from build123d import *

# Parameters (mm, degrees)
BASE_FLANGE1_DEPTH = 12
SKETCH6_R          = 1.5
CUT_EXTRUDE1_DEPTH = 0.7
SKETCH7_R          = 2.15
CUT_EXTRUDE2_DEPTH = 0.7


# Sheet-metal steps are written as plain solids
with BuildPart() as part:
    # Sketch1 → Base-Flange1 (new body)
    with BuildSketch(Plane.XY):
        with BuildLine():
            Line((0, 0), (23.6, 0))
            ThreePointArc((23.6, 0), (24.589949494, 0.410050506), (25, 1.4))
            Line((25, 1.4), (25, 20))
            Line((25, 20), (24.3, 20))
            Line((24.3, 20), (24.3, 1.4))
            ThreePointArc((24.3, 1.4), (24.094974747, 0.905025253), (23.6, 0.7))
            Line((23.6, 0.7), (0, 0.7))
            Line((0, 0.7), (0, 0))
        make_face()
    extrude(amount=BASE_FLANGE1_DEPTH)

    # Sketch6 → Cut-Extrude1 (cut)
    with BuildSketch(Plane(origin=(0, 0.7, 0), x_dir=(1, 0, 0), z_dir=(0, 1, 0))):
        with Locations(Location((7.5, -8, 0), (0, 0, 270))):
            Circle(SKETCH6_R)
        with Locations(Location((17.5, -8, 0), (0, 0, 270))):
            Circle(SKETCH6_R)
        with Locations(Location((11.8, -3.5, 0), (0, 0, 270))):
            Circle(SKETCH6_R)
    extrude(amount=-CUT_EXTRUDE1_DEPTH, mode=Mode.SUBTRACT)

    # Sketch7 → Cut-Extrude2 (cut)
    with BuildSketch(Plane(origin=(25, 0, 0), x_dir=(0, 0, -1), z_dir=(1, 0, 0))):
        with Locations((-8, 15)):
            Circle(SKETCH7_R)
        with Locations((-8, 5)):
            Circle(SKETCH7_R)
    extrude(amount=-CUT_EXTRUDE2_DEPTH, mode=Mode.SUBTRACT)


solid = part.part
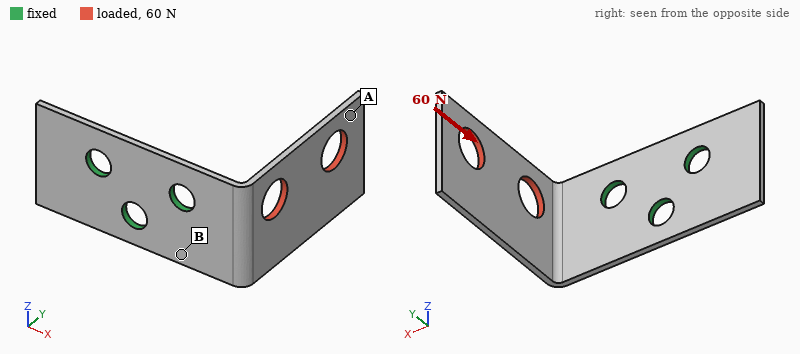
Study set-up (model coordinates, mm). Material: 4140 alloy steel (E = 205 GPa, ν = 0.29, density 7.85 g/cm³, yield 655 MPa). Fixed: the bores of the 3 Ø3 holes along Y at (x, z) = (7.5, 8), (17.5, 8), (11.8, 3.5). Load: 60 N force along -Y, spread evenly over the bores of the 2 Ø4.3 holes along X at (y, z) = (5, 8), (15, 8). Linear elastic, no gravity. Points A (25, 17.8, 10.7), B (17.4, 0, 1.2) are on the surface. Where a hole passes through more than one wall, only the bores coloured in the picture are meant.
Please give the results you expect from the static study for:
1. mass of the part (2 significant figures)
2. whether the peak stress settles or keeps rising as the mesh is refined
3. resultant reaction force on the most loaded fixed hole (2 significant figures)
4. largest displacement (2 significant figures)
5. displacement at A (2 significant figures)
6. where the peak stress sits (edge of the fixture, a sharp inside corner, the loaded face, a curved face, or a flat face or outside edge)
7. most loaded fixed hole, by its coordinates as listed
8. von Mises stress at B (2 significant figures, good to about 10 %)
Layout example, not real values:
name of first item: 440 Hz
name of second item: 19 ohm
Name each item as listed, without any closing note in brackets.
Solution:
mass of the part: 2.6 g
whether the peak stress settles or keeps rising as the mesh is refined: keeps rising
resultant reaction force on the most loaded fixed hole: 71 N
largest displacement: 0.35 mm
displacement at A: 0.31 mm
where the peak stress sits: edge of the fixture
most loaded fixed hole, by its coordinates as listed: (17.5, 8)
von Mises stress at B: 110 MPa
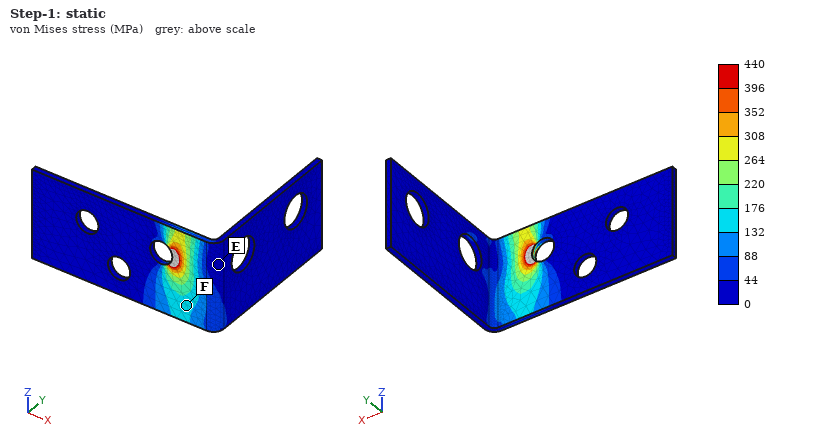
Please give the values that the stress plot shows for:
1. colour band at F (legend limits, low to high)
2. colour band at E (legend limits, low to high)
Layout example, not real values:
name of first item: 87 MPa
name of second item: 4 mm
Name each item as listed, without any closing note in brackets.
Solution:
colour band at F: 132 to 176 MPa
colour band at E: 0 to 44 MPa
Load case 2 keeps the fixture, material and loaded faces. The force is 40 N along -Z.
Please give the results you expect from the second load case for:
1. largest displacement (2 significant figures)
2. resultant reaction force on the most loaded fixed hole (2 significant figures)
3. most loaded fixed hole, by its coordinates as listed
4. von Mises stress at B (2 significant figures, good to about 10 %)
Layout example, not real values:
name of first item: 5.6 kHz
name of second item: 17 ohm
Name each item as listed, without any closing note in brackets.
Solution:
largest displacement: 0.38 mm
resultant reaction force on the most loaded fixed hole: 52 N
most loaded fixed hole, by its coordinates as listed: (17.5, 8)
von Mises stress at B: 190 MPa
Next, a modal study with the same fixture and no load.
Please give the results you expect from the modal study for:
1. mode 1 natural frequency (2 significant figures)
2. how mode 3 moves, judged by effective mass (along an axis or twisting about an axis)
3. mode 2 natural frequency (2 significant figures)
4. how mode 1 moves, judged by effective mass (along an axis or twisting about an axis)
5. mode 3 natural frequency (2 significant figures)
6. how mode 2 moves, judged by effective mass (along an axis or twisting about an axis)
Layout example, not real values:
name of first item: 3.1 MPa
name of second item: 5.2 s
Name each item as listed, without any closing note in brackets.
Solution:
mode 1 natural frequency: 1000 Hz
how mode 3 moves, judged by effective mass: along Y
mode 2 natural frequency: 1900 Hz
how mode 1 moves, judged by effective mass: along X
mode 3 natural frequency: 4700 Hz
how mode 2 moves, judged by effective mass: along Z
